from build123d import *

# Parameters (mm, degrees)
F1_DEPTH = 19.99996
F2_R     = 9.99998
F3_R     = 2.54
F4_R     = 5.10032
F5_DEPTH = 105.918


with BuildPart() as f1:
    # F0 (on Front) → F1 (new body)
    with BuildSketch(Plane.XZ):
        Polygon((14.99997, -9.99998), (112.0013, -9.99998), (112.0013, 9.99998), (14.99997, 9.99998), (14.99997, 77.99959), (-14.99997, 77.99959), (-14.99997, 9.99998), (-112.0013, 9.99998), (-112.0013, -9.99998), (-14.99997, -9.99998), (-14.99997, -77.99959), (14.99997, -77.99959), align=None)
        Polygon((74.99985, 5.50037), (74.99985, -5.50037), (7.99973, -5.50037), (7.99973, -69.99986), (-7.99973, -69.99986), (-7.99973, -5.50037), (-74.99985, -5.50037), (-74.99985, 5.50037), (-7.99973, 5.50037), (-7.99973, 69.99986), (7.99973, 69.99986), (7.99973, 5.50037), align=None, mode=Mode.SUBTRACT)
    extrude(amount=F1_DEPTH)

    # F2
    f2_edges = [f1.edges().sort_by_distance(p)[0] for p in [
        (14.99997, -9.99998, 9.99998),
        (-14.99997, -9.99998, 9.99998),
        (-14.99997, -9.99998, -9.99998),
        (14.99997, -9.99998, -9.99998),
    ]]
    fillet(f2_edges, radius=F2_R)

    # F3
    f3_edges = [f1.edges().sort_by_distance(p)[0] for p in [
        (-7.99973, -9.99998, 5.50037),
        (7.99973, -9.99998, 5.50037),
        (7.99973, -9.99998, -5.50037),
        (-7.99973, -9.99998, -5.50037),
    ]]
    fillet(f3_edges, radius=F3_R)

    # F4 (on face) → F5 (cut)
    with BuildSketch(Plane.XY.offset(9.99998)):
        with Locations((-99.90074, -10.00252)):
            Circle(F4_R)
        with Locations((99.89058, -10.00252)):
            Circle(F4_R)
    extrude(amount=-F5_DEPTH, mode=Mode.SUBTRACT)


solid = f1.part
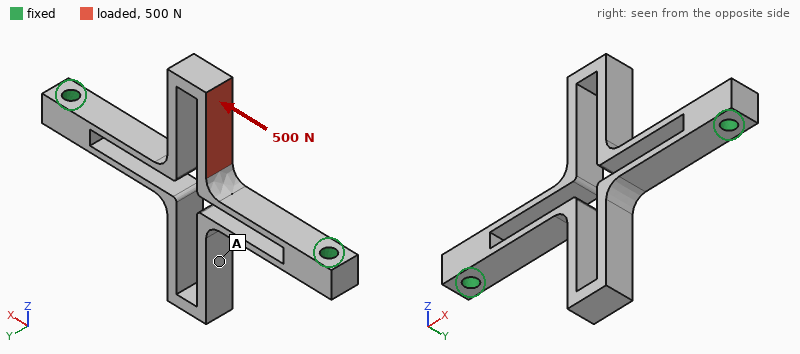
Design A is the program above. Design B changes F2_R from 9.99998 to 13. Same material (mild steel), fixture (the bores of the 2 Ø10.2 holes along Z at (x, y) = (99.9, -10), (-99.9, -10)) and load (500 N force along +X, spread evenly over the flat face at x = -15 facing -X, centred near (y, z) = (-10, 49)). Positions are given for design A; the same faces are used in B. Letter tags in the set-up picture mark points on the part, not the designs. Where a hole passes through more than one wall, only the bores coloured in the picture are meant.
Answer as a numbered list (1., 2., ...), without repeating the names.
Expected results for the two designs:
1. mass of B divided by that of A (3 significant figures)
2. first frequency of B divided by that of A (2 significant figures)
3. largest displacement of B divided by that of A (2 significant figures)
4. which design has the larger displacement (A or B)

1. 1.01
2. 1.0
3. 0.90
4. A
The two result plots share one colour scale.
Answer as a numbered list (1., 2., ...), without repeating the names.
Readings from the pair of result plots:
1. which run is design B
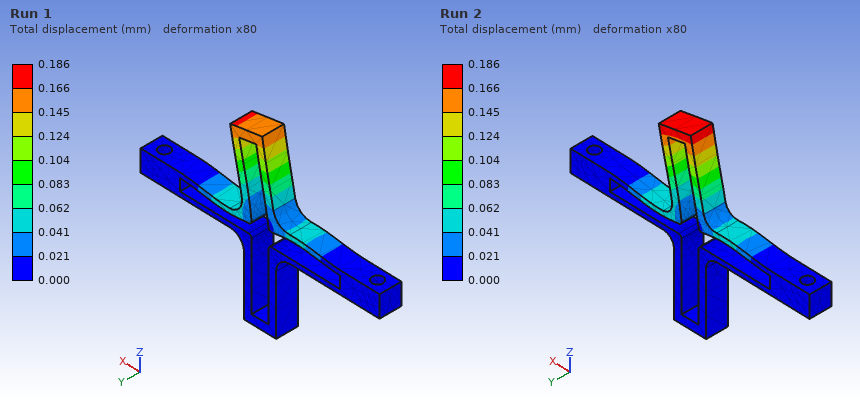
1. Run 1
